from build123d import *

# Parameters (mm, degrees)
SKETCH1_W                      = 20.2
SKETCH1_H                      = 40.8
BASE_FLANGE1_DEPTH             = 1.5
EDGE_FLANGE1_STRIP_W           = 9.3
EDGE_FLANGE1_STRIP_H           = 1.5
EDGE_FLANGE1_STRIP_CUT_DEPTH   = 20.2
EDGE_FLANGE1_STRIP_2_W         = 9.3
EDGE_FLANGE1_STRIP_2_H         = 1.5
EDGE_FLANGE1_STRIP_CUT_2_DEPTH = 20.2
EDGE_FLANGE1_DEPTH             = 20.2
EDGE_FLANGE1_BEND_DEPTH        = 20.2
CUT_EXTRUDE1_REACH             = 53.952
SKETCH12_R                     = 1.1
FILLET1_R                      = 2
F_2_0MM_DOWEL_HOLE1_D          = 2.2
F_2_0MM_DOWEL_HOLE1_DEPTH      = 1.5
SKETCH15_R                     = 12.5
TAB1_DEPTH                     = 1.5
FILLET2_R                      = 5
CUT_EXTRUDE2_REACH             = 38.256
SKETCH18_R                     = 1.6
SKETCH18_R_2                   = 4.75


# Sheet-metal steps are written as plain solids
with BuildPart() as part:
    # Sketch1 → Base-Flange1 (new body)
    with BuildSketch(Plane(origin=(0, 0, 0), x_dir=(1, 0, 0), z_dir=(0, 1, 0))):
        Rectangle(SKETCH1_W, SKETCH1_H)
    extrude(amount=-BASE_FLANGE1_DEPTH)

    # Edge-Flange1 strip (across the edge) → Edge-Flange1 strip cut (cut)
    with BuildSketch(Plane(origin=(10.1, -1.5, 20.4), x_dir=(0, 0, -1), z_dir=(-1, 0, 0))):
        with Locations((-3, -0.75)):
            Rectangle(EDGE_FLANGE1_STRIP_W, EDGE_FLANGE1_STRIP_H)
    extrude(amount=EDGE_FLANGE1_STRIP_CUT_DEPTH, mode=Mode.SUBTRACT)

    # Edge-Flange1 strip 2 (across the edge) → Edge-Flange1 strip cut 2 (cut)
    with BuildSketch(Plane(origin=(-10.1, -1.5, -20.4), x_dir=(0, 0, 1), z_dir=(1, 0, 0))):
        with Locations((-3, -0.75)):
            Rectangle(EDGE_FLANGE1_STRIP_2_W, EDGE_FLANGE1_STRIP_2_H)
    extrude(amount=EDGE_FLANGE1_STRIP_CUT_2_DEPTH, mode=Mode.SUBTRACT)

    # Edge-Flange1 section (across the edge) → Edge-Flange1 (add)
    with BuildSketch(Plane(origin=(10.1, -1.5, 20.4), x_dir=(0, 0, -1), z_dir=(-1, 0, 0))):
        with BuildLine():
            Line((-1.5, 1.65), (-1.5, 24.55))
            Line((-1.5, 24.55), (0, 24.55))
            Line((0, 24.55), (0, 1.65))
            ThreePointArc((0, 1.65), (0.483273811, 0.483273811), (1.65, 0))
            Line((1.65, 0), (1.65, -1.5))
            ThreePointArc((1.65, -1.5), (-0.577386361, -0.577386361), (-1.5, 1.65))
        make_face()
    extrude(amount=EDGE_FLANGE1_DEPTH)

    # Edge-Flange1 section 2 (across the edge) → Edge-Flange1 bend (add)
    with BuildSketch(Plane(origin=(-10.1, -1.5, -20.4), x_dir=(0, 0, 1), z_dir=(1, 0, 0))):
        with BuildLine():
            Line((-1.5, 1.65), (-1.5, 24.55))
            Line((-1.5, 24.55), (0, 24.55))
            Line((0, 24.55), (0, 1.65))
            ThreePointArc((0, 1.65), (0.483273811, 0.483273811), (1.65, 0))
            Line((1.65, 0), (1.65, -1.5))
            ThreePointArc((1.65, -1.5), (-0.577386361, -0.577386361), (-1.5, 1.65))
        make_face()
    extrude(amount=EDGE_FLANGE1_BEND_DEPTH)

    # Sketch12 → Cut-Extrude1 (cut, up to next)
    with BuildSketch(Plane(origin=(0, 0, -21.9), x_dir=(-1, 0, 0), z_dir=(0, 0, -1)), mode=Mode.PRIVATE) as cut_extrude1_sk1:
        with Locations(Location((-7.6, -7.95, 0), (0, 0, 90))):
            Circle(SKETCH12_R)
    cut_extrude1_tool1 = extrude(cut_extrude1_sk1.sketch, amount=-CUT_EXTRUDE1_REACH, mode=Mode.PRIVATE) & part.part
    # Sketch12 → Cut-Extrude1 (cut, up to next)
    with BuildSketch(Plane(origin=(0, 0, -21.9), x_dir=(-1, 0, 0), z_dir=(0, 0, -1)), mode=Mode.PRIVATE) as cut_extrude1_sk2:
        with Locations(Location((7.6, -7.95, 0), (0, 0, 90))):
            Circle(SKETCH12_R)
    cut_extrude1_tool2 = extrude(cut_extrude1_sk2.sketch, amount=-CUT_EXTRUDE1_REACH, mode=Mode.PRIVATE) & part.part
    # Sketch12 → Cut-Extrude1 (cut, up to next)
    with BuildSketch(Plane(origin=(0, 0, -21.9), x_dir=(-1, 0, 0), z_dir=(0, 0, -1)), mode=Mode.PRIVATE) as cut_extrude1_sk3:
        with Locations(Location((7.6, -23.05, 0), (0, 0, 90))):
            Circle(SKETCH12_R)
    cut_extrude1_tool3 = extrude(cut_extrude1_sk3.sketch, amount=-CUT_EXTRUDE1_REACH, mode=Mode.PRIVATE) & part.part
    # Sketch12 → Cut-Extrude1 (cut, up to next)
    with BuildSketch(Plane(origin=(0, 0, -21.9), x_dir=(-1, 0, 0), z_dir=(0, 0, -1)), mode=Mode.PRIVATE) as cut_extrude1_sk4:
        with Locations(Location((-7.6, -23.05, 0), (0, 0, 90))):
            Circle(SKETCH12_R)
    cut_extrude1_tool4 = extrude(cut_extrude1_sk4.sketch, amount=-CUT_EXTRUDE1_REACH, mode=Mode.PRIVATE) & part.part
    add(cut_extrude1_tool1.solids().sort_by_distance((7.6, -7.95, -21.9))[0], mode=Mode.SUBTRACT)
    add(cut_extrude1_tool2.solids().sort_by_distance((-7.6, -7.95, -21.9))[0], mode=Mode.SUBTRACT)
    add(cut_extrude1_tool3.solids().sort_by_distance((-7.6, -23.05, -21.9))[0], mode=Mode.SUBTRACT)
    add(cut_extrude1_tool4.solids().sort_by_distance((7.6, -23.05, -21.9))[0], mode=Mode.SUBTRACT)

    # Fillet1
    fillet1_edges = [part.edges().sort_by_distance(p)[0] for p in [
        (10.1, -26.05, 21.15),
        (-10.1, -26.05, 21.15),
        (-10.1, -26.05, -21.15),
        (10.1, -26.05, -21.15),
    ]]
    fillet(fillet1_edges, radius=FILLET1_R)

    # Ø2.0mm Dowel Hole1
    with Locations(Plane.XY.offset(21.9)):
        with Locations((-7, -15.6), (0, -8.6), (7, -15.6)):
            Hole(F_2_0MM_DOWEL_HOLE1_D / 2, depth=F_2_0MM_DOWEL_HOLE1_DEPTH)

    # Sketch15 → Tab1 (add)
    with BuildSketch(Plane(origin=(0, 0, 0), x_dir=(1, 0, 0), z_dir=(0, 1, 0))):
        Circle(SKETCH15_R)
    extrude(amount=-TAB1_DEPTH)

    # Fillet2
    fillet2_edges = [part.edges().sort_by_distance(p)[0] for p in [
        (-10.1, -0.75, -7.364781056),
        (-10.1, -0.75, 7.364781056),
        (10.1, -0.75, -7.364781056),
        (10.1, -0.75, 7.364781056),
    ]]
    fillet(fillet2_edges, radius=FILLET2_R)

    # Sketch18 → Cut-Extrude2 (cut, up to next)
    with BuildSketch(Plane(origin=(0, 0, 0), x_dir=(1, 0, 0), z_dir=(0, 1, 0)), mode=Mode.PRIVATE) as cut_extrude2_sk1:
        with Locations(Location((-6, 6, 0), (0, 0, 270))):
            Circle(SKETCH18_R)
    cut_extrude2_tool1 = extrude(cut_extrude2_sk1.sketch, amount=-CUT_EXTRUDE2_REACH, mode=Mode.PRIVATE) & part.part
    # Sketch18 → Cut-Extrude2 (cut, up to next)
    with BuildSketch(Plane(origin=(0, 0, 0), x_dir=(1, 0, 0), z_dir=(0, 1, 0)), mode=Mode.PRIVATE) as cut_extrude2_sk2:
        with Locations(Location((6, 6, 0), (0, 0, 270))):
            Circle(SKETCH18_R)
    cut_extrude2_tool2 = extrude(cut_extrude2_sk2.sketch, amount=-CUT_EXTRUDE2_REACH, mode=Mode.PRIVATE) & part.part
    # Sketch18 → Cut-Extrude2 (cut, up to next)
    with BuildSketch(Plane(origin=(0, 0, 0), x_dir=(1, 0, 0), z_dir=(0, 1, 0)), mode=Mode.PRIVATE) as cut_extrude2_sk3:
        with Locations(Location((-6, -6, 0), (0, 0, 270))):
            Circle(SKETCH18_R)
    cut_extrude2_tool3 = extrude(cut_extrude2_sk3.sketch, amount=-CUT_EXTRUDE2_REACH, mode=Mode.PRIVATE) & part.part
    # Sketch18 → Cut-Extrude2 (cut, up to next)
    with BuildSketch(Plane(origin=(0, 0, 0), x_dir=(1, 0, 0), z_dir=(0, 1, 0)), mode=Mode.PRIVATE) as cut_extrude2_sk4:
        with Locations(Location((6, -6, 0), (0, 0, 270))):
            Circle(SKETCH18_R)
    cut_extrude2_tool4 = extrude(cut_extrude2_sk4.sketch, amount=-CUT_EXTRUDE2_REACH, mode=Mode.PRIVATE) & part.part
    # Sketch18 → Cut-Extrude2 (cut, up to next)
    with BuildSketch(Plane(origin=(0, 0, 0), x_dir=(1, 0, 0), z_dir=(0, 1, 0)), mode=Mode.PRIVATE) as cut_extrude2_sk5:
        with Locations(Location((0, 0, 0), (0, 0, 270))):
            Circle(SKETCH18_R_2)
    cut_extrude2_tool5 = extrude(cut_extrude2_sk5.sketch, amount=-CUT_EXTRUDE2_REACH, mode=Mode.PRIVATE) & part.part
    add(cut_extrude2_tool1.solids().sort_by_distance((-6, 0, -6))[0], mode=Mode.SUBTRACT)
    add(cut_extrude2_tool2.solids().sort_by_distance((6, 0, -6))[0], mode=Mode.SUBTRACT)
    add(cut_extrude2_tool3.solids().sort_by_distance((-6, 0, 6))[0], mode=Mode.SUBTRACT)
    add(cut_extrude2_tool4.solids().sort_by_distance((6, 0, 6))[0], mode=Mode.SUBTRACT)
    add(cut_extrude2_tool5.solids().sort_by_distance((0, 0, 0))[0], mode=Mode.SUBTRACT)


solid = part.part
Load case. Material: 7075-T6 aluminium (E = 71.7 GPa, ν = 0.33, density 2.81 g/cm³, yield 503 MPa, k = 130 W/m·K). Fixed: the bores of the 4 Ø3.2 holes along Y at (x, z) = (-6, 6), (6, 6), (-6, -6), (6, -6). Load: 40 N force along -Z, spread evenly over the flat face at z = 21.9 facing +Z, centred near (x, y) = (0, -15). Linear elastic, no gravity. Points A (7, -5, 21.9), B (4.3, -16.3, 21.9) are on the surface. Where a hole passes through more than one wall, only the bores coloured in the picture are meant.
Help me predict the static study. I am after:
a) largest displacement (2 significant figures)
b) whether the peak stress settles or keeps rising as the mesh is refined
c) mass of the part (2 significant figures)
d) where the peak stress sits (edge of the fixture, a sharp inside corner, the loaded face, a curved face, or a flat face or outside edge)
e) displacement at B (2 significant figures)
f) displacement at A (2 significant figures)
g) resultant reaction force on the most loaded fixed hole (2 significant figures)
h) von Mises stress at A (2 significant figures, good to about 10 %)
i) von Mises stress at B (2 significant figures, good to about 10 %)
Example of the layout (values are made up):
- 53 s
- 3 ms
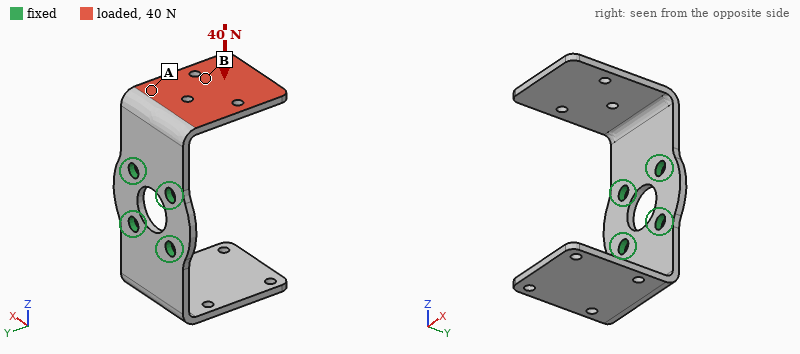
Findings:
- 0.66 mm
- keeps rising
- 7.4 g
- edge of the fixture
- 0.39 mm
- 0.17 mm
- 21 N
- 46 MPa
- 13 MPa
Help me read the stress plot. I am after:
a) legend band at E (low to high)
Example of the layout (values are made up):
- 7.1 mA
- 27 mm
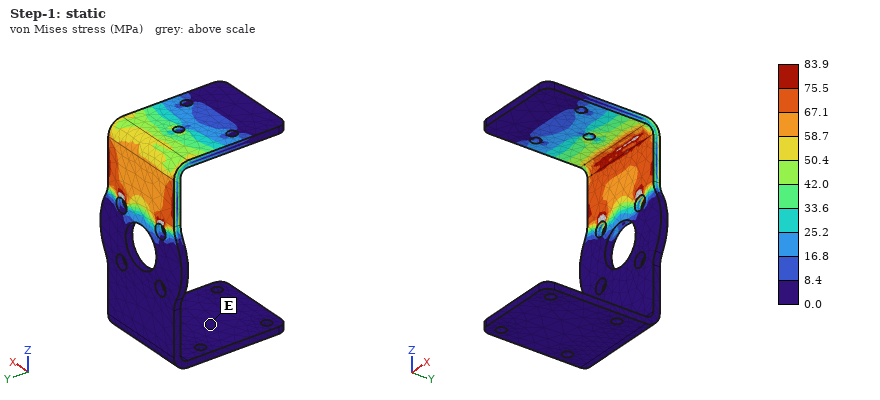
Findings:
- 0.0 to 8.4 MPa
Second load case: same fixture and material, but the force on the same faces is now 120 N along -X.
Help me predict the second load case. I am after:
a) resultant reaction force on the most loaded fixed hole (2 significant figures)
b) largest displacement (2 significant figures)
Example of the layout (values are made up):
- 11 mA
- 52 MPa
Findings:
- 180 N
- 0.55 mm
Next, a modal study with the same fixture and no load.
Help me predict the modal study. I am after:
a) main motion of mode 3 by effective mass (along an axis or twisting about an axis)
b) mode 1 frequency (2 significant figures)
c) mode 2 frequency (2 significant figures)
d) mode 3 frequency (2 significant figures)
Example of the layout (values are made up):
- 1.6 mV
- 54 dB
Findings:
- along X
- 1000 Hz
- 1100 Hz
- 1900 Hz
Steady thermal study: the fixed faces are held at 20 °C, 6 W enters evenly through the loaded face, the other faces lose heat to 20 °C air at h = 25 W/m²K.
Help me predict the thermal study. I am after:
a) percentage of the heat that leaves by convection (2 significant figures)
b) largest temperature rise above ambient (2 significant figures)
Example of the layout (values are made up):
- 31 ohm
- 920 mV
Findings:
- 11 %
- 39 K
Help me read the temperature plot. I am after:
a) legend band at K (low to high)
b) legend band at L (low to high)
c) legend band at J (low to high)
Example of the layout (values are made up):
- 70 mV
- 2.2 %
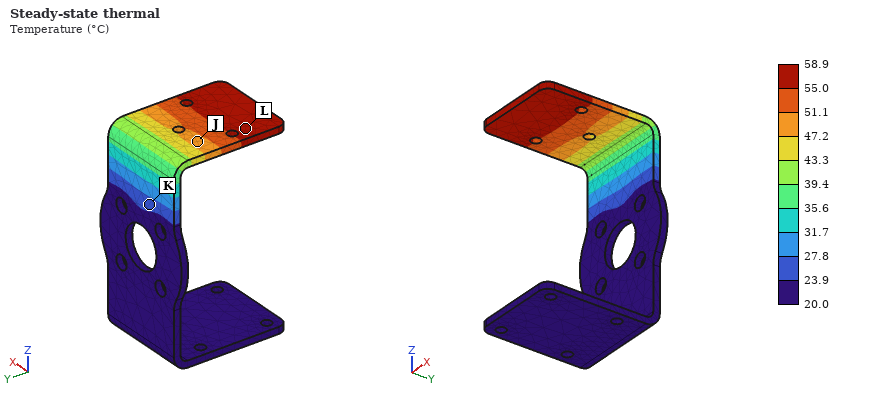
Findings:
- 23.9 to 27.8 °C
- 55.0 to 58.9 °C
- 47.2 to 51.1 °C
